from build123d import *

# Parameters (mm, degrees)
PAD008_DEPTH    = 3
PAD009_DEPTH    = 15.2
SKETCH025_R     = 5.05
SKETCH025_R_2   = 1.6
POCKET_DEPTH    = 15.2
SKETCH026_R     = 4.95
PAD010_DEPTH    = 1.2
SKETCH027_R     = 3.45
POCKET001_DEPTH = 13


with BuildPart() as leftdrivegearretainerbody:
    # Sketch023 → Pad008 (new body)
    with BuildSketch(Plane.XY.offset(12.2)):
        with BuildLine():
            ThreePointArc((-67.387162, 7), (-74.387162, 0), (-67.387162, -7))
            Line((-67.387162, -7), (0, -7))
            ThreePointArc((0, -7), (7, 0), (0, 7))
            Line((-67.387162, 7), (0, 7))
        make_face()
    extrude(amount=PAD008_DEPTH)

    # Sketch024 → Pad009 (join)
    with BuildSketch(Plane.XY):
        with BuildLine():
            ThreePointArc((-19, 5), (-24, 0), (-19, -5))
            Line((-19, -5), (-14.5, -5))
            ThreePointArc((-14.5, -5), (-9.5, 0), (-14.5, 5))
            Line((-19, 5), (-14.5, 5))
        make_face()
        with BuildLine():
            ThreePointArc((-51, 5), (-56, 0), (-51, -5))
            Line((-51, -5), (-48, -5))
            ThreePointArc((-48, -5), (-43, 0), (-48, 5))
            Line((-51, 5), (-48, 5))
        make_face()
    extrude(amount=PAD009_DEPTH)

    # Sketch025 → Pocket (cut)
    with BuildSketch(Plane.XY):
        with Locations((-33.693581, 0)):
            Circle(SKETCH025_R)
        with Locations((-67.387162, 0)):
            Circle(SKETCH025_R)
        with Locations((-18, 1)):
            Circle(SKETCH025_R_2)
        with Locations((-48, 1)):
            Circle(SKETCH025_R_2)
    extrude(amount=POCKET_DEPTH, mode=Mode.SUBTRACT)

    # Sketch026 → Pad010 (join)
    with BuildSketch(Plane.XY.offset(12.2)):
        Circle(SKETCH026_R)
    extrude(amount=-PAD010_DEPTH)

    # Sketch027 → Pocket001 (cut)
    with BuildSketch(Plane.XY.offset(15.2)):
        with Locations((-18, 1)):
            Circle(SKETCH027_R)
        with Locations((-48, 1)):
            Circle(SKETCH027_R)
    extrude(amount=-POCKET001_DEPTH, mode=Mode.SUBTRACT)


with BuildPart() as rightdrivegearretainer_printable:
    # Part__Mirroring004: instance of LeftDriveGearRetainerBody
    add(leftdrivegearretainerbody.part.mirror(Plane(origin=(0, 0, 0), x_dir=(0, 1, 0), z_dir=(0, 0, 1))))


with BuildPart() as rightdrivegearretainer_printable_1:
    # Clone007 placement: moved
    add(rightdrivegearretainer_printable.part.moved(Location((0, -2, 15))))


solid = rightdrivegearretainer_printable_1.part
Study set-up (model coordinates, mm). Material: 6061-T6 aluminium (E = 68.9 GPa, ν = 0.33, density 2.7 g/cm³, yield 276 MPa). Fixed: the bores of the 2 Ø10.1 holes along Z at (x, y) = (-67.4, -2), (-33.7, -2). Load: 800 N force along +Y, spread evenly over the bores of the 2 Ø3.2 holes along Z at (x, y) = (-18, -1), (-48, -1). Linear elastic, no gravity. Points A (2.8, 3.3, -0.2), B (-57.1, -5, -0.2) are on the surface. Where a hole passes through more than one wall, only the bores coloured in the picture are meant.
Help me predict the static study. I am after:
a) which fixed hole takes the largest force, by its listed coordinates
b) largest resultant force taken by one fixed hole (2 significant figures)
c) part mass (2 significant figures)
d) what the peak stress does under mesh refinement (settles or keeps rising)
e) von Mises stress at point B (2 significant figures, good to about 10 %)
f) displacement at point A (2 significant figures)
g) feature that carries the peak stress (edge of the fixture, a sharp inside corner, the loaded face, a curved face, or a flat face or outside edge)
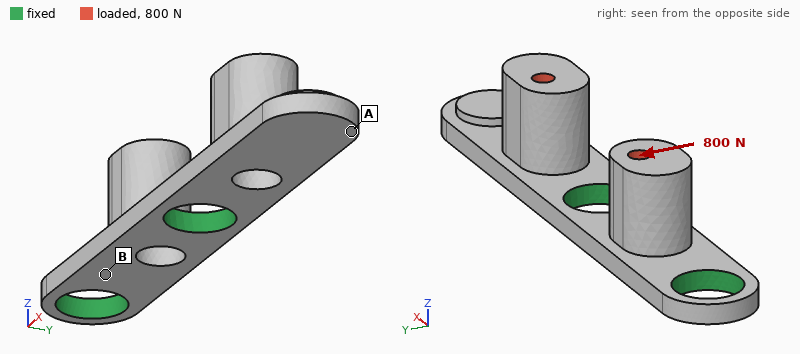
(-33.7, -2)
640 N
13 g
keeps rising
56 MPa
0.051 mm
edge of the fixture
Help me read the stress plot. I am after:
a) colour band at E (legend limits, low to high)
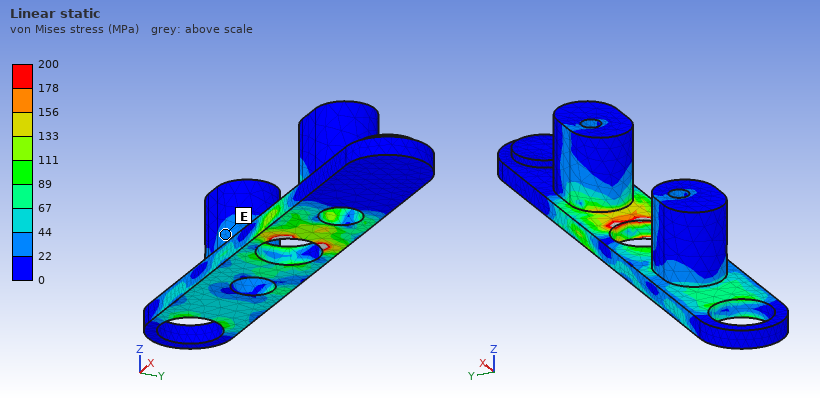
22 to 44 MPa
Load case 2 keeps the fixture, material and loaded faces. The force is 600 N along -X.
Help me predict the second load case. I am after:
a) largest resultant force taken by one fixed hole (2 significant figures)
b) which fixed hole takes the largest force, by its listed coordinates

480 N
(-33.7, -2)
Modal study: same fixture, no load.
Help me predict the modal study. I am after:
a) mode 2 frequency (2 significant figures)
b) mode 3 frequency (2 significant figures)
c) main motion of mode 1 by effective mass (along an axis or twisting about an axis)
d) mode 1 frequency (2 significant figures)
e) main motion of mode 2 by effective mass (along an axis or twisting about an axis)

5600 Hz
7100 Hz
along Z
1900 Hz
along Y
